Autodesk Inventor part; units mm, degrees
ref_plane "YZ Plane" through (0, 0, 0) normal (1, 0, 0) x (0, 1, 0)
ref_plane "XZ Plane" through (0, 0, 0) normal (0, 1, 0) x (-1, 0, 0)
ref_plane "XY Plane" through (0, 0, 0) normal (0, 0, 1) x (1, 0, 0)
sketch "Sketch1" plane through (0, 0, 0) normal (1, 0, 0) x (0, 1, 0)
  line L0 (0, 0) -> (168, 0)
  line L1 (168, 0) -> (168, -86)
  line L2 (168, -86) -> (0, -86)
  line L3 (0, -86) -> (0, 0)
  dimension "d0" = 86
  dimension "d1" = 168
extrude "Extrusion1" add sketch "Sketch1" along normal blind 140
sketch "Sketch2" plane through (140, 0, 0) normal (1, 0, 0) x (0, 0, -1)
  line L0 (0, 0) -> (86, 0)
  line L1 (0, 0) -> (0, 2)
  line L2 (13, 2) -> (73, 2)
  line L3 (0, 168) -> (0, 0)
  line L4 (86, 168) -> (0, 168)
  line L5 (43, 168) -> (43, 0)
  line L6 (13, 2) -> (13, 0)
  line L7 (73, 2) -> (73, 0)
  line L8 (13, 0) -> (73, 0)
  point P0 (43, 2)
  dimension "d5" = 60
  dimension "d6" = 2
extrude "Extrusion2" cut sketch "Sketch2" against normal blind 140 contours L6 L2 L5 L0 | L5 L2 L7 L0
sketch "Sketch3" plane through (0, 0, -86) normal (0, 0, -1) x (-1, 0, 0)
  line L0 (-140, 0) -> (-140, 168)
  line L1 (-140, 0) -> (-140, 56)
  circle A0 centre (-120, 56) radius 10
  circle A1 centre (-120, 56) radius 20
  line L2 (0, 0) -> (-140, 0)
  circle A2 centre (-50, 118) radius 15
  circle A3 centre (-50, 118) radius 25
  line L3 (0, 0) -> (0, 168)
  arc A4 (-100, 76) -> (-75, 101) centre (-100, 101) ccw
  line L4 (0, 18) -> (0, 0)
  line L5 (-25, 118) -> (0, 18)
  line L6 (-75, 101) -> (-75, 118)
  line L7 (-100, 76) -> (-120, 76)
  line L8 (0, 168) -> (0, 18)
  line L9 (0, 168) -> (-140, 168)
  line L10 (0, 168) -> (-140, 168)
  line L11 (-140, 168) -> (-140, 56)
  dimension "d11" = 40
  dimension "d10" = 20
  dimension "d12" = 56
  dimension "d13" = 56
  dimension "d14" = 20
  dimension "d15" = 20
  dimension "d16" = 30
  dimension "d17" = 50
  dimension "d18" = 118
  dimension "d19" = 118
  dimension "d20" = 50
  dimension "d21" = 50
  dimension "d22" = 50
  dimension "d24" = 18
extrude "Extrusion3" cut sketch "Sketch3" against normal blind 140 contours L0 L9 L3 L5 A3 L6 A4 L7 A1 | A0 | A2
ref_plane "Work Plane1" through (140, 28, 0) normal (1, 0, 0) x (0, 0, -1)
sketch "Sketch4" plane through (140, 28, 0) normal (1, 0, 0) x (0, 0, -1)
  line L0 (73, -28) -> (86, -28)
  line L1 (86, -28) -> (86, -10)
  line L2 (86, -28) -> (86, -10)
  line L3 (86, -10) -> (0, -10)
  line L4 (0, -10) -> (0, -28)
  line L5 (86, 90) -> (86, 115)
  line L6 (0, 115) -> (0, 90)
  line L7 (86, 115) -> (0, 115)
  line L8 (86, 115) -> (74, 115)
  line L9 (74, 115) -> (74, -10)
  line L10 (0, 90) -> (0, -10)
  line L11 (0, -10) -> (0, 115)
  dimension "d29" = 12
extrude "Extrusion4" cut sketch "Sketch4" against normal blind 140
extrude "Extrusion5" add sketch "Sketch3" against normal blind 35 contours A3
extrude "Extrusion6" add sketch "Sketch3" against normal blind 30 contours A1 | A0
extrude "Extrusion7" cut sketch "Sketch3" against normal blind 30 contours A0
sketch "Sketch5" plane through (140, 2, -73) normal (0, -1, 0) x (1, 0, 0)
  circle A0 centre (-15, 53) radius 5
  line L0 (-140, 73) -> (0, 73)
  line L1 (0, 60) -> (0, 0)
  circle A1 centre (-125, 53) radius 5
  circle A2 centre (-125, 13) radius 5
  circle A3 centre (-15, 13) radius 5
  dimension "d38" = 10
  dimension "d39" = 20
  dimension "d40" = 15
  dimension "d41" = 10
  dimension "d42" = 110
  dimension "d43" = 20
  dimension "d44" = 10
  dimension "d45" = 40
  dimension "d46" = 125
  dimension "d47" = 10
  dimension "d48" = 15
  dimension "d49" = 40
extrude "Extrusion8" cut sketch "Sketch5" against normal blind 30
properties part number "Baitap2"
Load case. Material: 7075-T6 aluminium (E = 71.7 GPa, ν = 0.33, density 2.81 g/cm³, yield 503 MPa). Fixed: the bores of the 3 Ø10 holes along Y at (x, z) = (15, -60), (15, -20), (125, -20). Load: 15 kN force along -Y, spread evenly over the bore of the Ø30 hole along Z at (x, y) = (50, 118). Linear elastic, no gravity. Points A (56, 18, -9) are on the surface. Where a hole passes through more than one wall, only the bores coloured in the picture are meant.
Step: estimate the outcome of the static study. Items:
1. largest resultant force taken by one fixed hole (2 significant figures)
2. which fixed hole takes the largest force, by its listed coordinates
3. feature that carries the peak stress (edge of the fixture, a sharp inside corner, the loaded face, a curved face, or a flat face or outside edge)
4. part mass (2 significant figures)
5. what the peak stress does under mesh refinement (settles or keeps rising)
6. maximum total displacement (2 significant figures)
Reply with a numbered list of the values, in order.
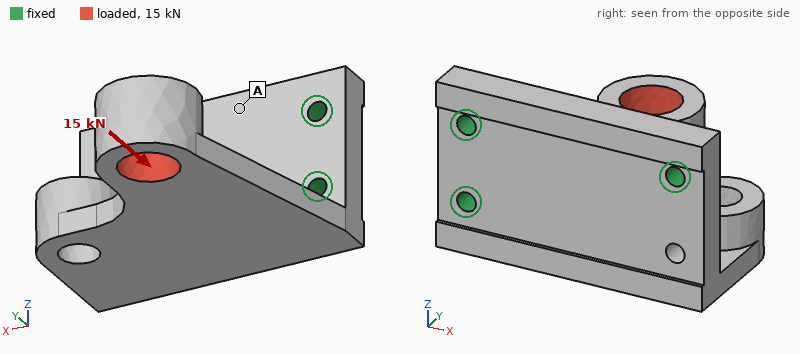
1. 12 kN
2. (15, -60)
3. edge of the fixture
4. 1.0 kg
5. keeps rising
6. 1.3 mm
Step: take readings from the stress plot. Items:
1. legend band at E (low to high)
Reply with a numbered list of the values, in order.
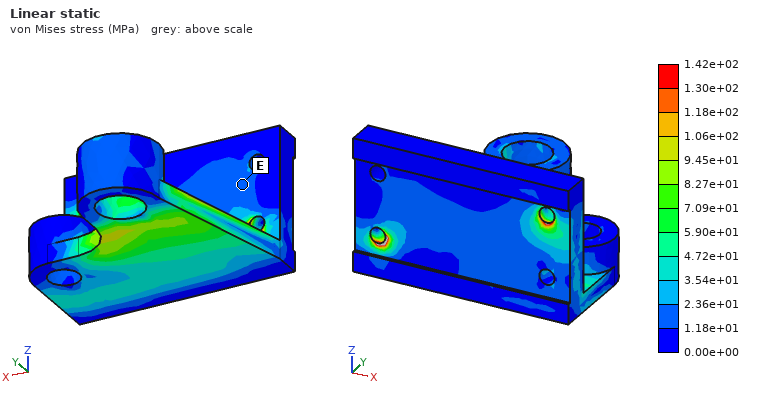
1. 1.18e+01 to 2.36e+01 MPa
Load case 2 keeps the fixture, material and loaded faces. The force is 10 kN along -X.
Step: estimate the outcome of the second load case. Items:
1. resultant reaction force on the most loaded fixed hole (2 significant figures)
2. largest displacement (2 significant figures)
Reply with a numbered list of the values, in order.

1. 9.1 kN
2. 0.97 mm
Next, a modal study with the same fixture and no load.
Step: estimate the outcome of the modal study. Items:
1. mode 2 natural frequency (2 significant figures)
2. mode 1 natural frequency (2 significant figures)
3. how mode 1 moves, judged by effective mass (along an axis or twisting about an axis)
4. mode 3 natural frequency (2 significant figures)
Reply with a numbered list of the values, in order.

1. 1200 Hz
2. 580 Hz
3. along Z
4. 2300 Hz
